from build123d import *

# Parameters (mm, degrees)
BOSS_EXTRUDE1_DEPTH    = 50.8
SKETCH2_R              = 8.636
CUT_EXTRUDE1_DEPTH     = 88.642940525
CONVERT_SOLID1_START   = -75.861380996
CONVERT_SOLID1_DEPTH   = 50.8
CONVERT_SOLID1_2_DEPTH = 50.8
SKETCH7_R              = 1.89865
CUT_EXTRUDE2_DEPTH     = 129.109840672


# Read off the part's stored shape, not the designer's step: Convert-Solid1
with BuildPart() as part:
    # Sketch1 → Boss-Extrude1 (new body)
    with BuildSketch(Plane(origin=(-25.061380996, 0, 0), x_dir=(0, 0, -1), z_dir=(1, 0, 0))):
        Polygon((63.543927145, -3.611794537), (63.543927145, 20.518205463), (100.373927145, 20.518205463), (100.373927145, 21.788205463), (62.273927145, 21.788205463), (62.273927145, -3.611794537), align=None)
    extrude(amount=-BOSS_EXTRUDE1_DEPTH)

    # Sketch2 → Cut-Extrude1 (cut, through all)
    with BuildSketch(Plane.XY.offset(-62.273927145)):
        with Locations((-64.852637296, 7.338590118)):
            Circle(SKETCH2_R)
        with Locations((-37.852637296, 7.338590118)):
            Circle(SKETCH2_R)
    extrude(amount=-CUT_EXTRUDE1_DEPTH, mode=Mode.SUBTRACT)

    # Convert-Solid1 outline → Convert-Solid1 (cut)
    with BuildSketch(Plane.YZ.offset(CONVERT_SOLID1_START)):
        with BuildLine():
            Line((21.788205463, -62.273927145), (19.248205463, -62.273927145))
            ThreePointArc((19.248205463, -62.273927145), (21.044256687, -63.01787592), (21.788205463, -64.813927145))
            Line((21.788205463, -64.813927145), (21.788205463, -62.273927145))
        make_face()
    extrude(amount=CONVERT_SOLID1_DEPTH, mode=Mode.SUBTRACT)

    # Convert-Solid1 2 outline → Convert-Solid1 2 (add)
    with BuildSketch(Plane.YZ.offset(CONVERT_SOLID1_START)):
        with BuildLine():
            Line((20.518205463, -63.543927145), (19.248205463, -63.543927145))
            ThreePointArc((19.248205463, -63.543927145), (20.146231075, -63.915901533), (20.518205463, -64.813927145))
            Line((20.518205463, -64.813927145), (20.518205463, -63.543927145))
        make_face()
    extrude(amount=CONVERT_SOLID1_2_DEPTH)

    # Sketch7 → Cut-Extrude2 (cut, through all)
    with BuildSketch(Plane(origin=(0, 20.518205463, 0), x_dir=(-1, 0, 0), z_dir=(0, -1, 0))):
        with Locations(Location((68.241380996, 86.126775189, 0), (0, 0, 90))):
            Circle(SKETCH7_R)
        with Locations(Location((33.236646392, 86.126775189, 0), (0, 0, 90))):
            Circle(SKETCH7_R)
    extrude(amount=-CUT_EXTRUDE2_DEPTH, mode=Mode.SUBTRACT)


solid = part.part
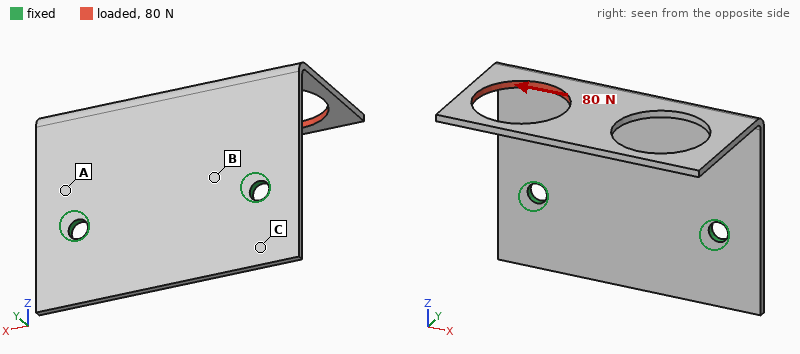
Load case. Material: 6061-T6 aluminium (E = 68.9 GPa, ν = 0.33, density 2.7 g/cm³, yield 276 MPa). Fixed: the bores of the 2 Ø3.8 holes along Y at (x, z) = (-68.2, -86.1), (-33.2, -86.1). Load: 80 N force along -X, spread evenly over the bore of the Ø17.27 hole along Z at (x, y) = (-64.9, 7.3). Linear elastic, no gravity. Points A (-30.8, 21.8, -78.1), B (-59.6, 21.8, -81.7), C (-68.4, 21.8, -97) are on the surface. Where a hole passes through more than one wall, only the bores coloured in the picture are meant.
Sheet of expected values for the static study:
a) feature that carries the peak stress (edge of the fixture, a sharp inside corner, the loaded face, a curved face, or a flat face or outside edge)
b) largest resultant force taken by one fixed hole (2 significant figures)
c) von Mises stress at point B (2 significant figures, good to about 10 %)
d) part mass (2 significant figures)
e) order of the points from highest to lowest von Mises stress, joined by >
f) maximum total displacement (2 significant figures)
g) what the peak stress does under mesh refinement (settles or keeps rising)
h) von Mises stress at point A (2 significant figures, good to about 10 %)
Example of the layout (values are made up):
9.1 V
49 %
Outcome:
edge of the fixture
71 N
22 MPa
9.0 g
A > B > C
0.43 mm
keeps rising
39 MPa
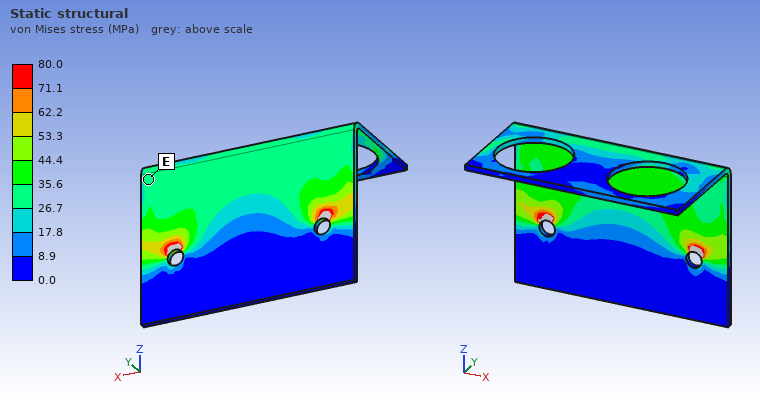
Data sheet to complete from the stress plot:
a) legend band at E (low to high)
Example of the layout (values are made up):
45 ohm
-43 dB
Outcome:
26.7 to 35.6 MPa
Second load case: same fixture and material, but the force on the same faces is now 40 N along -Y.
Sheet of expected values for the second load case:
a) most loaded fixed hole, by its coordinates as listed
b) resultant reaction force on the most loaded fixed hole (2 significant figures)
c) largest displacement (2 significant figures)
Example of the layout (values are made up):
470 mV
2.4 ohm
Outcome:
(-68.2, -86.1)
35 N
0.70 mm
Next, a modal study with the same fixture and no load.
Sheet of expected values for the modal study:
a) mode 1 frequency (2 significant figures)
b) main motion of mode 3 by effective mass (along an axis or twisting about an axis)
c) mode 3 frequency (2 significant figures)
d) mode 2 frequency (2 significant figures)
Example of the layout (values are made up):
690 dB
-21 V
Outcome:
740 Hz
along Y
1700 Hz
1300 Hz
